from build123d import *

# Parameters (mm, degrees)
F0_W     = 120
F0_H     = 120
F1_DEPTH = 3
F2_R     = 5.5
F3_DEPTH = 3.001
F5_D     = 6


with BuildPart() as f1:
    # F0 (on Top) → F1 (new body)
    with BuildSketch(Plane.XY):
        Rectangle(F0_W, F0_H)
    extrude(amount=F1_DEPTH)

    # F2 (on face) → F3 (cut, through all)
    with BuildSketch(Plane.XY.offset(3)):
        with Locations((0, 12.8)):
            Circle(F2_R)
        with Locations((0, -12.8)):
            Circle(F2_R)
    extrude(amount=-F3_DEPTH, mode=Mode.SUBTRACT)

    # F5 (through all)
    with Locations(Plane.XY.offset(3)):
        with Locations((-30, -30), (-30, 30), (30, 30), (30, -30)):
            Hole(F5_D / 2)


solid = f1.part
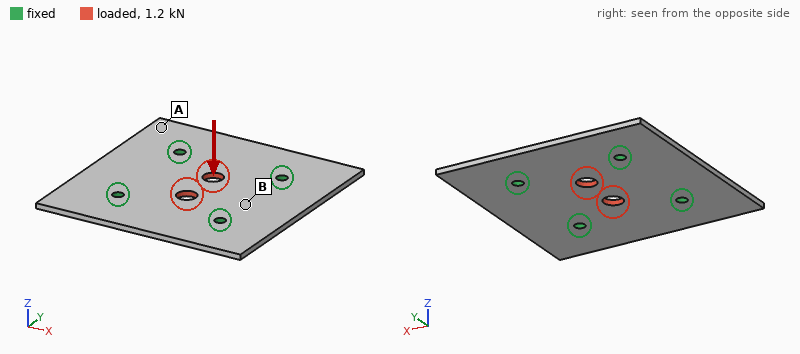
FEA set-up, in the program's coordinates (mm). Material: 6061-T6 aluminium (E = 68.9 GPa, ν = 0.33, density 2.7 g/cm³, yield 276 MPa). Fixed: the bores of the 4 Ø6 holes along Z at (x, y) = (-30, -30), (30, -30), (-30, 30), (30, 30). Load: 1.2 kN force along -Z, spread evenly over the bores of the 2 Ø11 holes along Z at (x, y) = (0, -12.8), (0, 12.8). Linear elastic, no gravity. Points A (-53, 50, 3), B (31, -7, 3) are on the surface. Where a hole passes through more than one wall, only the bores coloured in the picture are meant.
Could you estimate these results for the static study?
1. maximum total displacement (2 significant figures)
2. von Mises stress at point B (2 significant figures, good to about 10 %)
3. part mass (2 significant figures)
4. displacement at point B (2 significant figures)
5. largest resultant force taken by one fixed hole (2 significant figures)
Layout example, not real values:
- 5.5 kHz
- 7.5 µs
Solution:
- 0.27 mm
- 34 MPa
- 110 g
- 0.049 mm
- 300 N
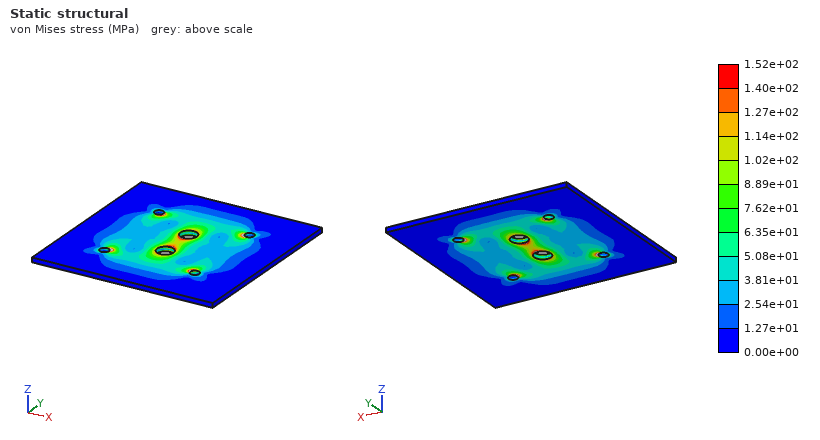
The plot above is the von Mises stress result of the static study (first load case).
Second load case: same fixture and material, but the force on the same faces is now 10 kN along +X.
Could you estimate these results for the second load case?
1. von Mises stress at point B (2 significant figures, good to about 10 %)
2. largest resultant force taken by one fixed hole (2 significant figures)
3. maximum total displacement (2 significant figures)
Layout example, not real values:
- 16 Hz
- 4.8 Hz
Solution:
- 15 MPa
- 2.6 kN
- 24 µm
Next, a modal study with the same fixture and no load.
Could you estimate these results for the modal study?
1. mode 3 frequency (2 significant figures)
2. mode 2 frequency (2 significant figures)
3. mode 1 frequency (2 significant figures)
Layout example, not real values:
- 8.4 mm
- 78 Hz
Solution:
- 2300 Hz
- 2200 Hz
- 2200 Hz
